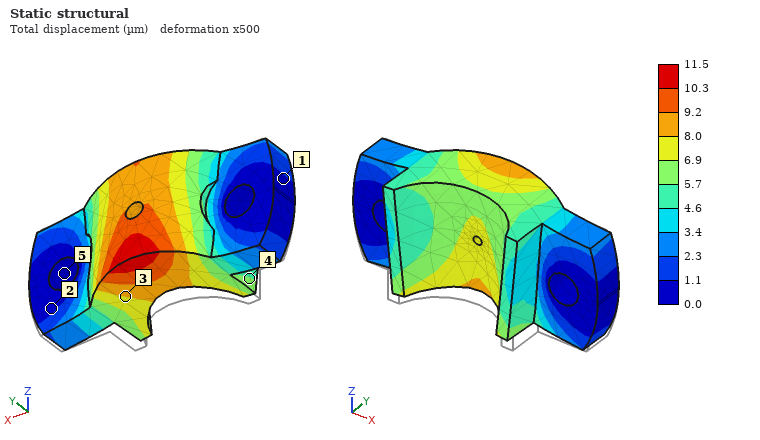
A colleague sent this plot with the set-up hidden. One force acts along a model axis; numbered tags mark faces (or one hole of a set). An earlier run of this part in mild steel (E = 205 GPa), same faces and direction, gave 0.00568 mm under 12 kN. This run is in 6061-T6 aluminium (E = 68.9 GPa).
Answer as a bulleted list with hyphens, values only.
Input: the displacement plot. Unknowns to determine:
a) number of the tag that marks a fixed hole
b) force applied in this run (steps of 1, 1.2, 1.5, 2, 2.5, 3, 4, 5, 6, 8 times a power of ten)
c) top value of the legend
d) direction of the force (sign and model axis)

- 5
- 8 kN
- 11.5 µm
- +Z
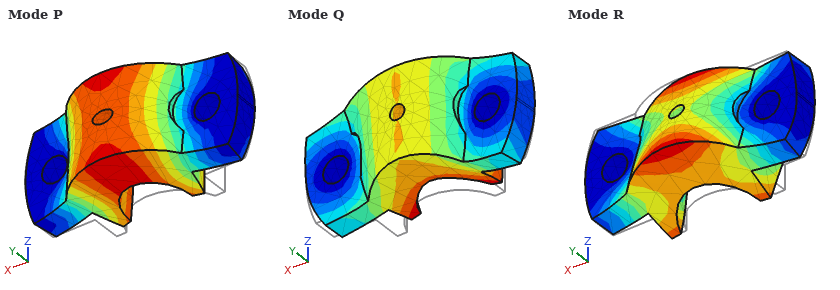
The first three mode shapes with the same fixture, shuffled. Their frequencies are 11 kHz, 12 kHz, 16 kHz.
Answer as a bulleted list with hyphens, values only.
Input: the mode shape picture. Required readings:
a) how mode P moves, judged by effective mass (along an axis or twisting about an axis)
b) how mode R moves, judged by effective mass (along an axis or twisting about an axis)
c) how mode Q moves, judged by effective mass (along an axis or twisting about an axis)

- along Y
- twisting about X
- along Z
